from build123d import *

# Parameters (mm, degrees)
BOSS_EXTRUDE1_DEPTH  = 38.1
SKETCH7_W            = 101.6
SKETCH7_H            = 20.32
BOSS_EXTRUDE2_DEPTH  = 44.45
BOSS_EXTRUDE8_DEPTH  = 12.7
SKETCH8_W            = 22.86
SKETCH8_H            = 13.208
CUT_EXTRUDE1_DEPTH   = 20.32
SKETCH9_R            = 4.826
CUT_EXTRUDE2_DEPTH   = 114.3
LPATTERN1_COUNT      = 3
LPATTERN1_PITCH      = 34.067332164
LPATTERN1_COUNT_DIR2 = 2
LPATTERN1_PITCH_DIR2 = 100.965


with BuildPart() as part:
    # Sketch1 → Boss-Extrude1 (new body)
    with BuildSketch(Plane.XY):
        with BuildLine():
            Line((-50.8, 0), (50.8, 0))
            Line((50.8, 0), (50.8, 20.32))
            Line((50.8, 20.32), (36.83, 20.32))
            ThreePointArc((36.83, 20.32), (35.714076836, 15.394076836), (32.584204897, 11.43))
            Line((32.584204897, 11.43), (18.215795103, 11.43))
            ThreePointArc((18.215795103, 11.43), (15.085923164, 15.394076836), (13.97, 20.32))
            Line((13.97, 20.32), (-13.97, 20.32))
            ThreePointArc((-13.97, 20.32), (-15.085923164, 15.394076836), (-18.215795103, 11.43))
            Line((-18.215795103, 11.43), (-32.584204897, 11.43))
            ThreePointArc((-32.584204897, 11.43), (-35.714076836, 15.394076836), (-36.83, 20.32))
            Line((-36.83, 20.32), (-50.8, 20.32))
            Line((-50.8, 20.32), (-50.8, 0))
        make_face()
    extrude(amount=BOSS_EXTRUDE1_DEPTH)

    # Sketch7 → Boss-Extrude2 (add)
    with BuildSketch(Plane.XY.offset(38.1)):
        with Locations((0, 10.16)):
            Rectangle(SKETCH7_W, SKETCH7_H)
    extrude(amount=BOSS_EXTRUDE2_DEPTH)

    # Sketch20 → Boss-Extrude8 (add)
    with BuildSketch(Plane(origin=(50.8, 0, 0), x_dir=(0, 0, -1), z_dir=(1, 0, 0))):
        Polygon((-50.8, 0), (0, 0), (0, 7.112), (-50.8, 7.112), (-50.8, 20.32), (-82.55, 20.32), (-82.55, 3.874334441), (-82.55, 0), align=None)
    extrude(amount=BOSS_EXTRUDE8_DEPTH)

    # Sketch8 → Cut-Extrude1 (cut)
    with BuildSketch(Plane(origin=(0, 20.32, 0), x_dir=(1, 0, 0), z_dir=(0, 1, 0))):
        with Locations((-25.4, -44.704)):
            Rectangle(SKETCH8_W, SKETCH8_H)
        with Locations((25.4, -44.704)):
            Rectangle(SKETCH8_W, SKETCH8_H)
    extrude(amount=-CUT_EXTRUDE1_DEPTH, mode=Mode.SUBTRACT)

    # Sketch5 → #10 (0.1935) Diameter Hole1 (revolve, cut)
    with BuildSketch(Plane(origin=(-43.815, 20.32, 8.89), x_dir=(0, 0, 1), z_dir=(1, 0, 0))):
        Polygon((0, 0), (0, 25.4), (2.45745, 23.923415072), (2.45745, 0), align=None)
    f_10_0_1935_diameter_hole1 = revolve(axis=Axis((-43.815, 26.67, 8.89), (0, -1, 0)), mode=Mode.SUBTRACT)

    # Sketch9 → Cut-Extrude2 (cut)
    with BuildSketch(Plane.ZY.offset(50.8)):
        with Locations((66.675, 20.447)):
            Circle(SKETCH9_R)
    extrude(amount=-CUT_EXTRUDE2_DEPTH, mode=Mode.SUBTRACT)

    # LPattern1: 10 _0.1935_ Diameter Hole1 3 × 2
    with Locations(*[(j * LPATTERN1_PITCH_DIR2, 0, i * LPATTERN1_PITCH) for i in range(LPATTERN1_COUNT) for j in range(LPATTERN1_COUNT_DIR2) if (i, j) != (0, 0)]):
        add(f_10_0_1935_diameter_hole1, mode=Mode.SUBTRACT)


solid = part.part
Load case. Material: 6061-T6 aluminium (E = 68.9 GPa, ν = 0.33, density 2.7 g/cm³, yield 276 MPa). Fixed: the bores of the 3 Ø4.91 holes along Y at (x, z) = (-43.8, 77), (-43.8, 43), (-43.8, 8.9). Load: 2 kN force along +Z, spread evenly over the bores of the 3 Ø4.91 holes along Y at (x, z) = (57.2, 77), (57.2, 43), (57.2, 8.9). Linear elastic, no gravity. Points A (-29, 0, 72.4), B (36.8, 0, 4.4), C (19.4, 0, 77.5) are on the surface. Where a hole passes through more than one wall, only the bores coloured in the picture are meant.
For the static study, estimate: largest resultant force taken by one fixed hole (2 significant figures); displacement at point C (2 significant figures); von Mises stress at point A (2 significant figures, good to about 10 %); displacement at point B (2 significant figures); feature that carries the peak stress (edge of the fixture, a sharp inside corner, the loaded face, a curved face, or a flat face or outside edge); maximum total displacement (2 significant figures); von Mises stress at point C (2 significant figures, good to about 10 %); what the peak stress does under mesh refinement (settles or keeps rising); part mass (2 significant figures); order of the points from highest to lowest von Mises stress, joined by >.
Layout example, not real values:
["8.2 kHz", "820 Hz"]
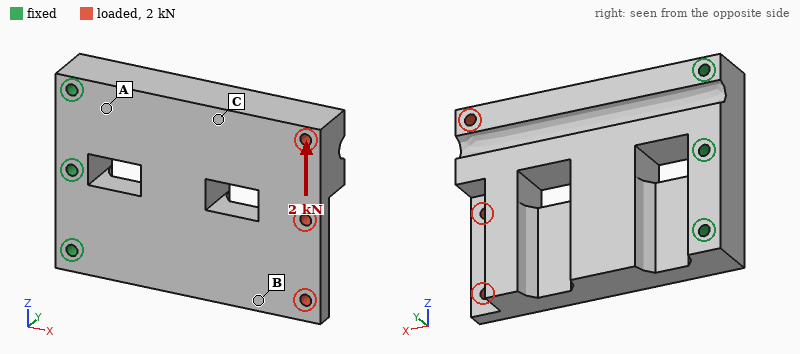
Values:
["3.0 kN", "19 µm", "11 MPa", "28 µm", "edge of the fixture", "41 µm", "5.9 MPa", "keeps rising", "410 g", "A > C > B"]
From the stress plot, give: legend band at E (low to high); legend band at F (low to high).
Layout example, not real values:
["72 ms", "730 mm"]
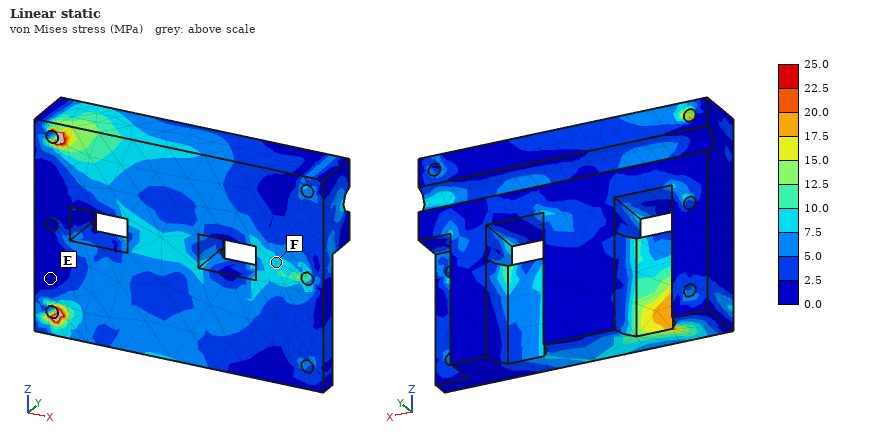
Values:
["0.0 to 2.5 MPa", "7.5 to 10.0 MPa"]
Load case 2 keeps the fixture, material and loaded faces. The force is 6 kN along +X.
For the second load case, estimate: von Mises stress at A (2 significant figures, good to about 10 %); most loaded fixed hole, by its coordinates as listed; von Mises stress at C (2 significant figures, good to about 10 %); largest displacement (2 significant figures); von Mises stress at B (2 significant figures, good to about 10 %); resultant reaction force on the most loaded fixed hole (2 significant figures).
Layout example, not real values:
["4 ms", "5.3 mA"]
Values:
["11 MPa", "(-43.8, 77)", "11 MPa", "35 µm", "7.8 MPa", "3.4 kN"]
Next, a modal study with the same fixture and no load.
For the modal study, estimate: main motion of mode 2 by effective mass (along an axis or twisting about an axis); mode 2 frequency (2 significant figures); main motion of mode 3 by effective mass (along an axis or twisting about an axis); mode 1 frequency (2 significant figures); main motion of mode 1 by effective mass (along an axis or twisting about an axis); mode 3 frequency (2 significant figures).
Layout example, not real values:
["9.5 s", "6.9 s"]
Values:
["twisting about X", "3000 Hz", "along Z", "1100 Hz", "along Y", "3900 Hz"]
